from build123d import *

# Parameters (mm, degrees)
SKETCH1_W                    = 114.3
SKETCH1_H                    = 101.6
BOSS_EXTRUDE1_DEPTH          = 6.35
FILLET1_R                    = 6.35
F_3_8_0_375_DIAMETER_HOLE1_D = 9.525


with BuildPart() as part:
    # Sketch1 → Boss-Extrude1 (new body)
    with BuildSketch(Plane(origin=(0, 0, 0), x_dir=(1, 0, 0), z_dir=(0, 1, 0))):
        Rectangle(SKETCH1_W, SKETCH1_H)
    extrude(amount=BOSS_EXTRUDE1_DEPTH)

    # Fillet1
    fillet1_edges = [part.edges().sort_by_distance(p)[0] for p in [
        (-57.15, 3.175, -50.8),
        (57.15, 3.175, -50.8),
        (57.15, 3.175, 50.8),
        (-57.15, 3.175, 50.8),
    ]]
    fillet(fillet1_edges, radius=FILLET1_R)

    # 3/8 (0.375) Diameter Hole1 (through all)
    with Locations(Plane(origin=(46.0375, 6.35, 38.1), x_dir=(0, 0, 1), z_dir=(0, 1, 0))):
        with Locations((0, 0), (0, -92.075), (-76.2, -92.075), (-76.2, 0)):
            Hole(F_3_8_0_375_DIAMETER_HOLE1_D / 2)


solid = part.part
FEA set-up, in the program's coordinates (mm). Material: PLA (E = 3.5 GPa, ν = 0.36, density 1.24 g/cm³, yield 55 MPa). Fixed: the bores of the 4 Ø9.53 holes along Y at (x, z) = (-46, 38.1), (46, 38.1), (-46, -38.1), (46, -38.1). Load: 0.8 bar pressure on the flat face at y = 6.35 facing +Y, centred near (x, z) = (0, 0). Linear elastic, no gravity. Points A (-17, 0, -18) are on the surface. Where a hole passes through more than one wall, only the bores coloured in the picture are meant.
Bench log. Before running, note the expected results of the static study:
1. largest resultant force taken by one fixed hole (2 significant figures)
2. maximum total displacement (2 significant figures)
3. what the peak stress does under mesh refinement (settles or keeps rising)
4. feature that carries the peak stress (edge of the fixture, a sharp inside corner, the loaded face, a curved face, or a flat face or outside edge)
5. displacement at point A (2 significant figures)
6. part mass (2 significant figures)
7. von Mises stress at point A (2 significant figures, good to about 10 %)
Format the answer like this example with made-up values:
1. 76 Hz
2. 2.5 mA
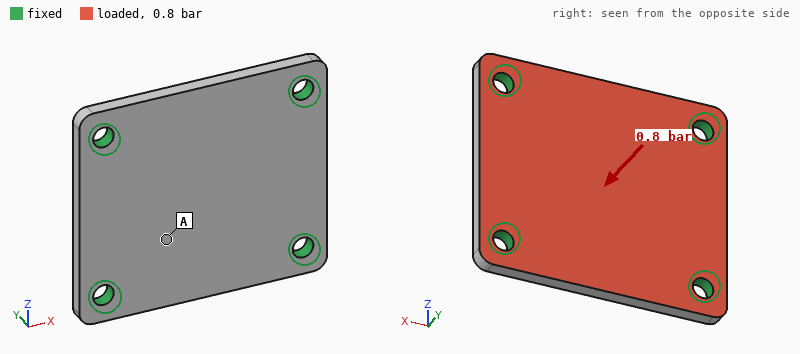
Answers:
1. 230 N
2. 0.30 mm
3. keeps rising
4. edge of the fixture
5. 0.22 mm
6. 89 g
7. 2.8 MPa
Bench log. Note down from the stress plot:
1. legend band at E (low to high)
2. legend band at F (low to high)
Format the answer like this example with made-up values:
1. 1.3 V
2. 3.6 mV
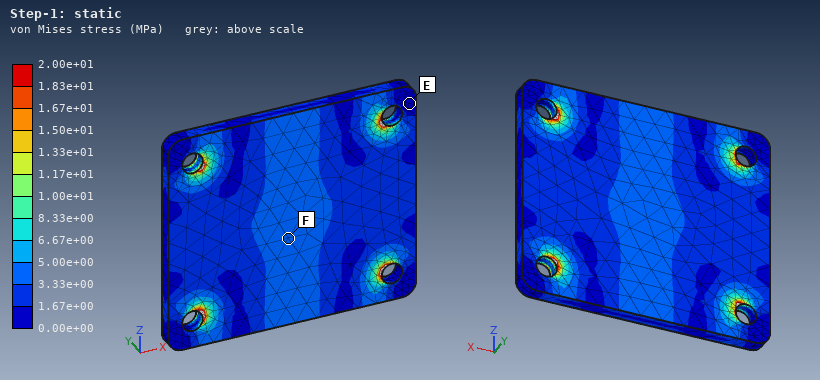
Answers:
1. 0.00e+00 to 1.67e+00 MPa
2. 3.33e+00 to 5.00e+00 MPa
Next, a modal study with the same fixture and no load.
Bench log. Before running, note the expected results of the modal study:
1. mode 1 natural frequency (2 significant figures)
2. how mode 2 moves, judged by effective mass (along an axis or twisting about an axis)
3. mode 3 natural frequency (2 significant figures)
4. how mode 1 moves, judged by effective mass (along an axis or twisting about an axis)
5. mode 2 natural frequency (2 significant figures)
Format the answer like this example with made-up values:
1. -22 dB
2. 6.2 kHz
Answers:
1. 1100 Hz
2. twisting about X
3. 1900 Hz
4. along Y
5. 1600 Hz
